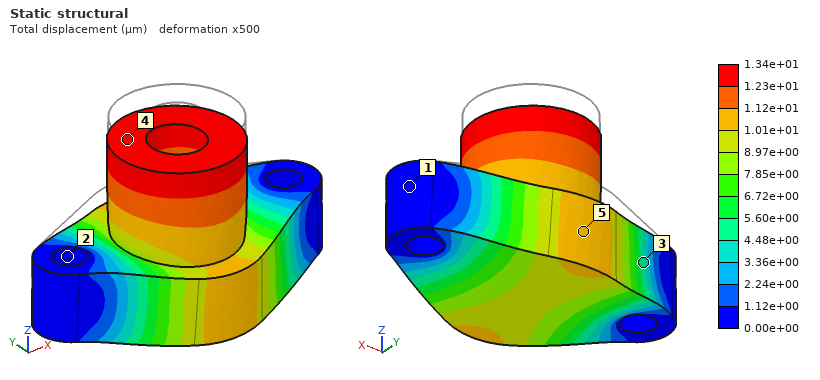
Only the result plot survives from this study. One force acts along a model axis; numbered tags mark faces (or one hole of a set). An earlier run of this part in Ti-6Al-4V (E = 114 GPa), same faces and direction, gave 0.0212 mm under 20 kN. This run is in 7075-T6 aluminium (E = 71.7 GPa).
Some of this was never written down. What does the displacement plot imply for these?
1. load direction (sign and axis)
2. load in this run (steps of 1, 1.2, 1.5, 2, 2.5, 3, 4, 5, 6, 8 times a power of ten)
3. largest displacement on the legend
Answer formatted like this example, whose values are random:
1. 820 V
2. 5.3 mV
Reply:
1. -Z
2. 8 kN
3. 1.34e+01 µm
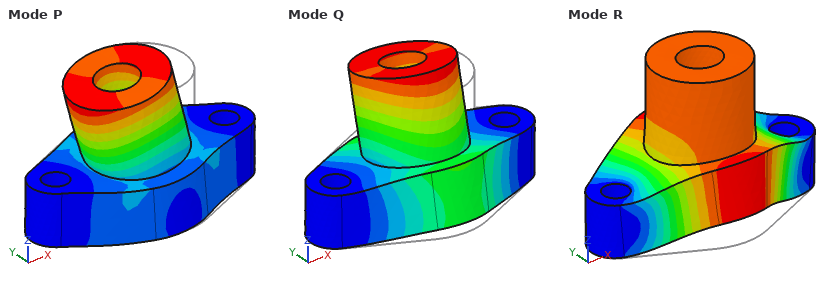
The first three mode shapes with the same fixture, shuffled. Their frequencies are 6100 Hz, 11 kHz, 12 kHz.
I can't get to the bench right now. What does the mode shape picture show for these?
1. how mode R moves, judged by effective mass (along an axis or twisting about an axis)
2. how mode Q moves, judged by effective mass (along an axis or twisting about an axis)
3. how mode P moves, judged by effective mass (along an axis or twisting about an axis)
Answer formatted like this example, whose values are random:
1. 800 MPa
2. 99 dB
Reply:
1. along Z
2. along Y
3. along X
